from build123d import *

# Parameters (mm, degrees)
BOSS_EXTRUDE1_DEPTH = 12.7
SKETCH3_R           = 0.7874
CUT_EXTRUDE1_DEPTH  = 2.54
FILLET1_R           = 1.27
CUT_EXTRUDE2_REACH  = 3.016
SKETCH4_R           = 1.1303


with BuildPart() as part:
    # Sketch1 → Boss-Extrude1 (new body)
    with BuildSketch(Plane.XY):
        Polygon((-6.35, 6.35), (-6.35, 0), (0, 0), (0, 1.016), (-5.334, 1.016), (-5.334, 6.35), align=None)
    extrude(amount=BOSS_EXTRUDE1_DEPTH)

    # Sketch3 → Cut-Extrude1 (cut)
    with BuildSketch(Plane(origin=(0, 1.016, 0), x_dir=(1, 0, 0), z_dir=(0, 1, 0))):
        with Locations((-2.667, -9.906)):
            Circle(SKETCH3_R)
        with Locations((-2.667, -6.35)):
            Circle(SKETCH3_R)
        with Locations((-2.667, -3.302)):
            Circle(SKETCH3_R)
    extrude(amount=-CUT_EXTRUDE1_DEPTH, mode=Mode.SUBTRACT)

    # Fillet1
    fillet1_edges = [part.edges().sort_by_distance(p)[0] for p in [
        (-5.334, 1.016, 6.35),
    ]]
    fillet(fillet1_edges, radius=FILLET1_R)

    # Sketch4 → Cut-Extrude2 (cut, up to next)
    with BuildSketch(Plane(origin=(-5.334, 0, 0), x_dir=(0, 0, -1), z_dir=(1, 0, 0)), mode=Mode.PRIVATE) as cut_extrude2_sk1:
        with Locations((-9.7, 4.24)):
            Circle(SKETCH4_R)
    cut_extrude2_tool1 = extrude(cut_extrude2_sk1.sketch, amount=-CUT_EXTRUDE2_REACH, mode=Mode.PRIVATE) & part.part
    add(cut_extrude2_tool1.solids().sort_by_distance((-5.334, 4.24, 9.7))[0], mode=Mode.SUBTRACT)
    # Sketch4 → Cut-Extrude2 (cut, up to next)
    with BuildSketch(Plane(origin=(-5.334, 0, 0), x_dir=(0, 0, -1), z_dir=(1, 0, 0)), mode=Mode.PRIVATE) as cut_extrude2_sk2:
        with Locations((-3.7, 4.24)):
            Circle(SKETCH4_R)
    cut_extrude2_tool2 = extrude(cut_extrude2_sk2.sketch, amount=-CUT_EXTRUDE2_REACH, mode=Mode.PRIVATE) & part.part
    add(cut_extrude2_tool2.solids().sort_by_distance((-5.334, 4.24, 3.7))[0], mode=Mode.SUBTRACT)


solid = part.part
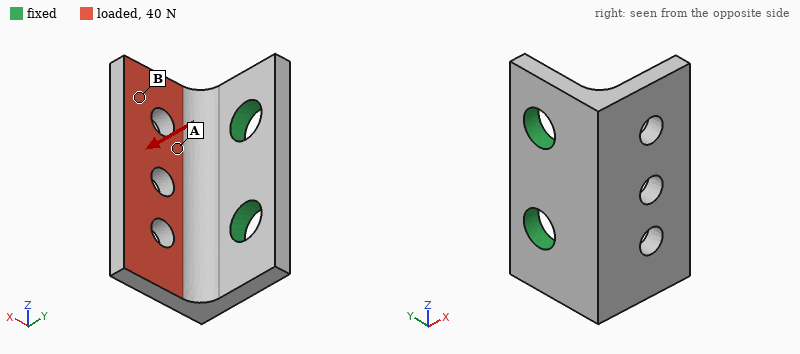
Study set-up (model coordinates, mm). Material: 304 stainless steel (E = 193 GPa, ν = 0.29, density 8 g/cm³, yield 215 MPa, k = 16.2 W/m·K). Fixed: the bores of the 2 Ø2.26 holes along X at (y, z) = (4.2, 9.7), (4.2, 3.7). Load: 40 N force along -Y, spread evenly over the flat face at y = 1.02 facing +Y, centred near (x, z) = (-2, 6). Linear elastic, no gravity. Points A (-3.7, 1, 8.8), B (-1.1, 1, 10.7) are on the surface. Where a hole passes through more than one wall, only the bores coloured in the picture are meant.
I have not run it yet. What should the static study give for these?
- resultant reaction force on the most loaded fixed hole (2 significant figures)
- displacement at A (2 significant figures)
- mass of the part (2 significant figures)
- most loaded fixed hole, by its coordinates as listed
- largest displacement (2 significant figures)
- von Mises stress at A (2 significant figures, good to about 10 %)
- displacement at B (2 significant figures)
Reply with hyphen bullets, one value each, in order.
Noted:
- 22 N
- 4.3 µm
- 1.1 g
- (4.2, 3.7)
- 14 µm
- 38 MPa
- 11 µm
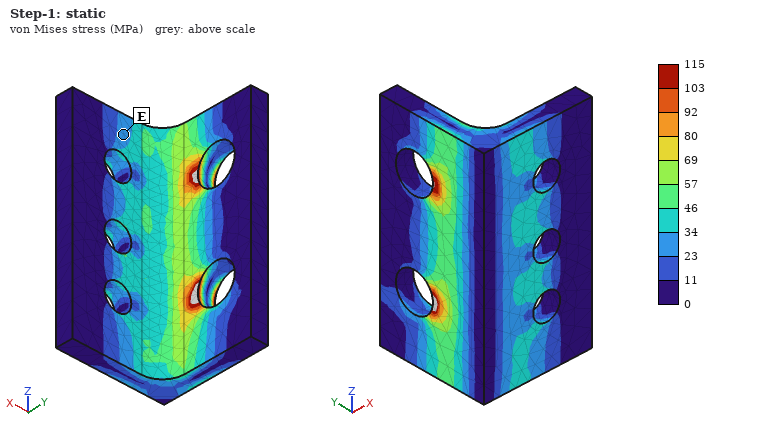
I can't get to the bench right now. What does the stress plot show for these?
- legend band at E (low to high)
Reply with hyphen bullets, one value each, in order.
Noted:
- 23 to 34 MPa
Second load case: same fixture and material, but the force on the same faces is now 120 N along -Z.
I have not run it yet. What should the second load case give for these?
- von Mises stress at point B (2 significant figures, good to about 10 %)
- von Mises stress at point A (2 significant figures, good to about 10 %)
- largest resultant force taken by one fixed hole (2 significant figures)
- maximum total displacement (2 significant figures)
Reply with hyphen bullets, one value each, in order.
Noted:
- 31 MPa
- 55 MPa
- 95 N
- 12 µm
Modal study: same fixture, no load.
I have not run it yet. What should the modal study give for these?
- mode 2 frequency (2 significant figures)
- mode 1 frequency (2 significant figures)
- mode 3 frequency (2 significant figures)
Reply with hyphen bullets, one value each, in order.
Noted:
- 24 kHz
- 15 kHz
- 40 kHz
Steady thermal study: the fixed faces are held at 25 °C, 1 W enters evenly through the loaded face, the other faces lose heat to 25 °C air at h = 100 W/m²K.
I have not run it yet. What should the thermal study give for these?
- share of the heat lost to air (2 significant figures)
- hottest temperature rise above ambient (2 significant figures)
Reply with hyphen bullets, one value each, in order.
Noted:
- 29 %
- 26 K
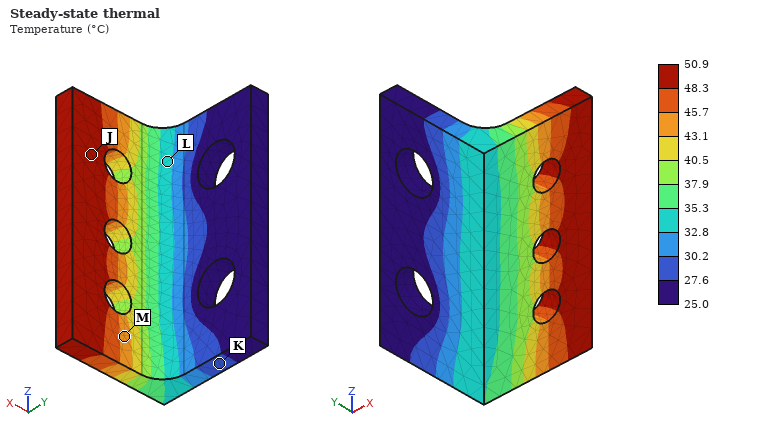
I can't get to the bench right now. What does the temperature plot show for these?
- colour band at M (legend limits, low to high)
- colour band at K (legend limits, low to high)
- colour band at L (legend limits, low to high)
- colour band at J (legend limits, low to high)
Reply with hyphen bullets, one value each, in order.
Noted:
- 43.1 to 45.7 °C
- 27.6 to 30.2 °C
- 32.8 to 35.3 °C
- 48.3 to 50.9 °C
